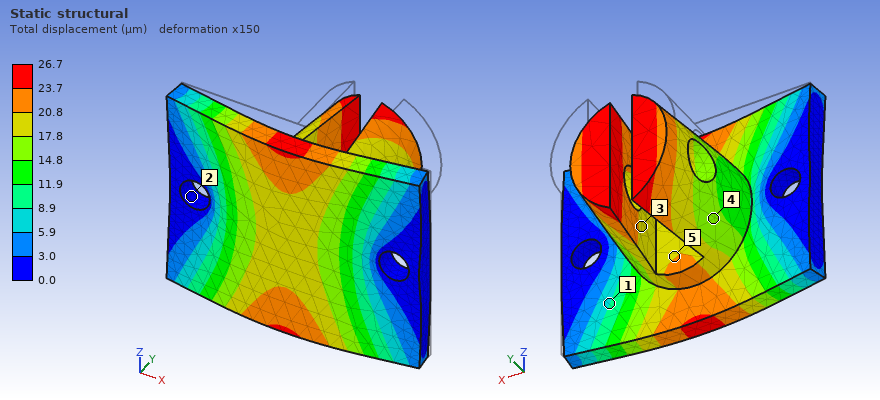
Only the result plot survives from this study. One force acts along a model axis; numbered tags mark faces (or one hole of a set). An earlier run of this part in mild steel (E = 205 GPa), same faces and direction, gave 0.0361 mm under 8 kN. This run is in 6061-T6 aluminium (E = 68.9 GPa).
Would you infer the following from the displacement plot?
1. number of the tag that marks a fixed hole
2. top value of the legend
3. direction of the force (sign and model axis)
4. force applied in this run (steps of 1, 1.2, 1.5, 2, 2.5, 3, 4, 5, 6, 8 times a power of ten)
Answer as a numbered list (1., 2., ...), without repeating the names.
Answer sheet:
1. 2
2. 26.7 µm
3. -Y
4. 2 kN
